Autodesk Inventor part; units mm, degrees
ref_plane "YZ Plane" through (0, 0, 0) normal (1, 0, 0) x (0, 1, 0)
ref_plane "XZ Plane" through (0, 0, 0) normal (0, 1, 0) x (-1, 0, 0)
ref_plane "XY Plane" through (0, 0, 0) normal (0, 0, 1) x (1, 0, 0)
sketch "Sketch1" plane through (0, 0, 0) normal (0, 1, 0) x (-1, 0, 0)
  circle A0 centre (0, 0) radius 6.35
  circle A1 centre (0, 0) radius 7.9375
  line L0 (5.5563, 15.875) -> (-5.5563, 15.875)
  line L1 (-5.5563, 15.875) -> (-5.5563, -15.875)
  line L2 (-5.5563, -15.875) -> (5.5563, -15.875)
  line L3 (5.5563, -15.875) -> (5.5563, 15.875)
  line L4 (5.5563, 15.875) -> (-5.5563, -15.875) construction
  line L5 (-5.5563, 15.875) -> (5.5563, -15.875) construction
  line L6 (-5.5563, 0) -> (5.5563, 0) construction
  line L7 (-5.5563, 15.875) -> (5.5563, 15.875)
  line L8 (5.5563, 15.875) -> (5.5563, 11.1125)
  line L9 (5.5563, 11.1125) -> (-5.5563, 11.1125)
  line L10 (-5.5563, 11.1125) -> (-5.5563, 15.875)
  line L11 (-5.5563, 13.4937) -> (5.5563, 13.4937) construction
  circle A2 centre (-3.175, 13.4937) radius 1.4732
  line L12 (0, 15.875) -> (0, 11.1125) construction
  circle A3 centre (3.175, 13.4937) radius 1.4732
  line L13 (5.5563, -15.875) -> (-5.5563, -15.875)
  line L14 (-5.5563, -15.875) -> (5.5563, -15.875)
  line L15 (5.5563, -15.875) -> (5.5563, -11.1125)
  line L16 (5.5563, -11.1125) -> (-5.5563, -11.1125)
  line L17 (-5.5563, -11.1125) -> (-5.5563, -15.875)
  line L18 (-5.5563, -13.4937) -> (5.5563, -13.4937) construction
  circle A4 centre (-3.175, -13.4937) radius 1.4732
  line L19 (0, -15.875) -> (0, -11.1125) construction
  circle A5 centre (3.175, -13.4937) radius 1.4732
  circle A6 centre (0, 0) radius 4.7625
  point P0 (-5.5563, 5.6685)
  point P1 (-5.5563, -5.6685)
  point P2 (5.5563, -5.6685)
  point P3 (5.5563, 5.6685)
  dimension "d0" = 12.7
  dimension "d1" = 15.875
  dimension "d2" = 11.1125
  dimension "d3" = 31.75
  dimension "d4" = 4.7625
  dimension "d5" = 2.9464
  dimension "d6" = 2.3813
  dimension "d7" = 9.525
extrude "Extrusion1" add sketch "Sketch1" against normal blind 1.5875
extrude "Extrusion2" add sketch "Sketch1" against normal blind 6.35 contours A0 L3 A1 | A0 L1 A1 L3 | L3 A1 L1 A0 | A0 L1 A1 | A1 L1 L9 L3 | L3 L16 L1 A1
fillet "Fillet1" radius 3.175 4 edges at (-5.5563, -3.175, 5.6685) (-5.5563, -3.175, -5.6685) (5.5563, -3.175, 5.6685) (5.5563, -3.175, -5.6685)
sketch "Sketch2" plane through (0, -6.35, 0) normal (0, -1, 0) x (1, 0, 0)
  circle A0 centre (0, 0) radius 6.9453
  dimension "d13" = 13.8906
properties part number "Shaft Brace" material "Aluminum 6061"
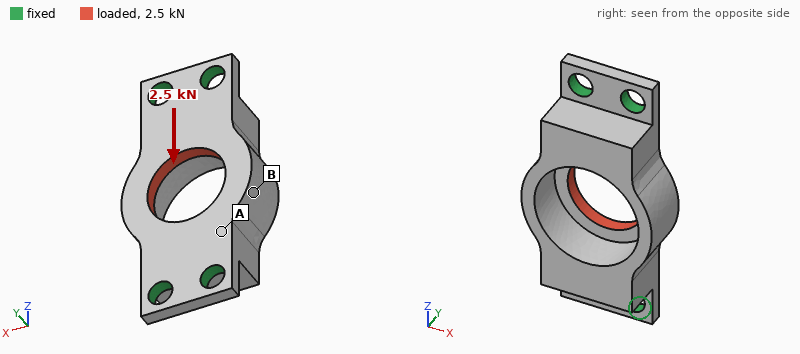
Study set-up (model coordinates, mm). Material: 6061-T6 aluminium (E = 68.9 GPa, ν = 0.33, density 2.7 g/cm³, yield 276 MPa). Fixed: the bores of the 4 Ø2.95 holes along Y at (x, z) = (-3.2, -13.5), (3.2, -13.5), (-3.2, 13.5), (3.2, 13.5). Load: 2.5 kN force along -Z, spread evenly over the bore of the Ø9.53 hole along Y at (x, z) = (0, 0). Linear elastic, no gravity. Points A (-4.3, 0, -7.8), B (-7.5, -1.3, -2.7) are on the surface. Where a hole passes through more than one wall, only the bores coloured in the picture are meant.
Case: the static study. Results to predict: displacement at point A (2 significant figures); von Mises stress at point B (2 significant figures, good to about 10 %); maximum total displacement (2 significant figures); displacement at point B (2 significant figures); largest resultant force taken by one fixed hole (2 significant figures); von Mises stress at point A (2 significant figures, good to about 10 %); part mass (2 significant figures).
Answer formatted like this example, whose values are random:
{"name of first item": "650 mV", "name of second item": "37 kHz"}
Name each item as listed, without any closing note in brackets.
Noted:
{"displacement at point A": "5.3 µm", "von Mises stress at point B": "19 MPa", "maximum total displacement": "12 µm", "displacement at point B": "8.1 µm", "largest resultant force taken by one fixed hole": "630 N", "von Mises stress at point A": "74 MPa", "part mass": "3.3 g"}
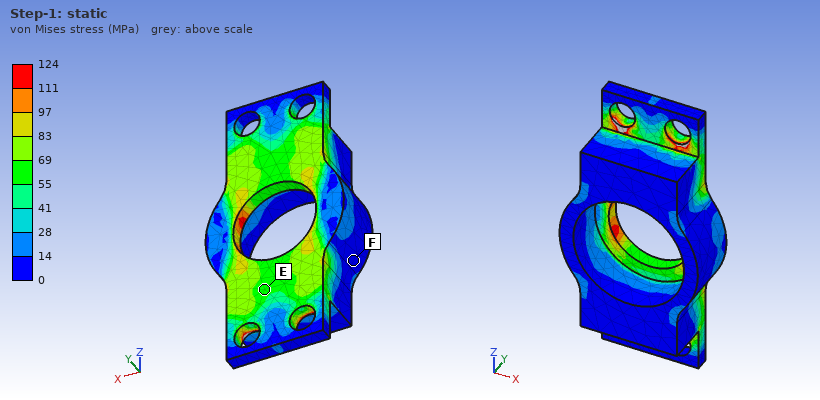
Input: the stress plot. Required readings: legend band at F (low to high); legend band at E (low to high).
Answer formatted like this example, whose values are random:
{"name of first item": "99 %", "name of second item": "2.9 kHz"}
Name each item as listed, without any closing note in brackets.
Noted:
{"legend band at F": "0 to 14 MPa", "legend band at E": "55 to 69 MPa"}
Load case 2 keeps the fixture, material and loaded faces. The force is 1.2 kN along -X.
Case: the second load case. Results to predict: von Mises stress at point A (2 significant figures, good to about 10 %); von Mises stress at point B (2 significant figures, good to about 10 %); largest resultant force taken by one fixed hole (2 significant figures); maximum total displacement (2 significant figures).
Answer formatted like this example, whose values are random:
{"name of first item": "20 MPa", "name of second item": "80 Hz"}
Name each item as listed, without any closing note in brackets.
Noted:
{"von Mises stress at point A": "35 MPa", "von Mises stress at point B": "38 MPa", "largest resultant force taken by one fixed hole": "400 N", "maximum total displacement": "18 µm"}
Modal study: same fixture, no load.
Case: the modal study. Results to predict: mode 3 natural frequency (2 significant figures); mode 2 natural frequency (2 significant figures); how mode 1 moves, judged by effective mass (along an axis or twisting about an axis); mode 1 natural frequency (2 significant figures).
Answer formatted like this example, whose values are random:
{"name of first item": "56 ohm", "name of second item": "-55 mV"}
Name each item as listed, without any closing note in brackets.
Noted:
{"mode 3 natural frequency": "40 kHz", "mode 2 natural frequency": "23 kHz", "how mode 1 moves, judged by effective mass": "along Y", "mode 1 natural frequency": "17 kHz"}
